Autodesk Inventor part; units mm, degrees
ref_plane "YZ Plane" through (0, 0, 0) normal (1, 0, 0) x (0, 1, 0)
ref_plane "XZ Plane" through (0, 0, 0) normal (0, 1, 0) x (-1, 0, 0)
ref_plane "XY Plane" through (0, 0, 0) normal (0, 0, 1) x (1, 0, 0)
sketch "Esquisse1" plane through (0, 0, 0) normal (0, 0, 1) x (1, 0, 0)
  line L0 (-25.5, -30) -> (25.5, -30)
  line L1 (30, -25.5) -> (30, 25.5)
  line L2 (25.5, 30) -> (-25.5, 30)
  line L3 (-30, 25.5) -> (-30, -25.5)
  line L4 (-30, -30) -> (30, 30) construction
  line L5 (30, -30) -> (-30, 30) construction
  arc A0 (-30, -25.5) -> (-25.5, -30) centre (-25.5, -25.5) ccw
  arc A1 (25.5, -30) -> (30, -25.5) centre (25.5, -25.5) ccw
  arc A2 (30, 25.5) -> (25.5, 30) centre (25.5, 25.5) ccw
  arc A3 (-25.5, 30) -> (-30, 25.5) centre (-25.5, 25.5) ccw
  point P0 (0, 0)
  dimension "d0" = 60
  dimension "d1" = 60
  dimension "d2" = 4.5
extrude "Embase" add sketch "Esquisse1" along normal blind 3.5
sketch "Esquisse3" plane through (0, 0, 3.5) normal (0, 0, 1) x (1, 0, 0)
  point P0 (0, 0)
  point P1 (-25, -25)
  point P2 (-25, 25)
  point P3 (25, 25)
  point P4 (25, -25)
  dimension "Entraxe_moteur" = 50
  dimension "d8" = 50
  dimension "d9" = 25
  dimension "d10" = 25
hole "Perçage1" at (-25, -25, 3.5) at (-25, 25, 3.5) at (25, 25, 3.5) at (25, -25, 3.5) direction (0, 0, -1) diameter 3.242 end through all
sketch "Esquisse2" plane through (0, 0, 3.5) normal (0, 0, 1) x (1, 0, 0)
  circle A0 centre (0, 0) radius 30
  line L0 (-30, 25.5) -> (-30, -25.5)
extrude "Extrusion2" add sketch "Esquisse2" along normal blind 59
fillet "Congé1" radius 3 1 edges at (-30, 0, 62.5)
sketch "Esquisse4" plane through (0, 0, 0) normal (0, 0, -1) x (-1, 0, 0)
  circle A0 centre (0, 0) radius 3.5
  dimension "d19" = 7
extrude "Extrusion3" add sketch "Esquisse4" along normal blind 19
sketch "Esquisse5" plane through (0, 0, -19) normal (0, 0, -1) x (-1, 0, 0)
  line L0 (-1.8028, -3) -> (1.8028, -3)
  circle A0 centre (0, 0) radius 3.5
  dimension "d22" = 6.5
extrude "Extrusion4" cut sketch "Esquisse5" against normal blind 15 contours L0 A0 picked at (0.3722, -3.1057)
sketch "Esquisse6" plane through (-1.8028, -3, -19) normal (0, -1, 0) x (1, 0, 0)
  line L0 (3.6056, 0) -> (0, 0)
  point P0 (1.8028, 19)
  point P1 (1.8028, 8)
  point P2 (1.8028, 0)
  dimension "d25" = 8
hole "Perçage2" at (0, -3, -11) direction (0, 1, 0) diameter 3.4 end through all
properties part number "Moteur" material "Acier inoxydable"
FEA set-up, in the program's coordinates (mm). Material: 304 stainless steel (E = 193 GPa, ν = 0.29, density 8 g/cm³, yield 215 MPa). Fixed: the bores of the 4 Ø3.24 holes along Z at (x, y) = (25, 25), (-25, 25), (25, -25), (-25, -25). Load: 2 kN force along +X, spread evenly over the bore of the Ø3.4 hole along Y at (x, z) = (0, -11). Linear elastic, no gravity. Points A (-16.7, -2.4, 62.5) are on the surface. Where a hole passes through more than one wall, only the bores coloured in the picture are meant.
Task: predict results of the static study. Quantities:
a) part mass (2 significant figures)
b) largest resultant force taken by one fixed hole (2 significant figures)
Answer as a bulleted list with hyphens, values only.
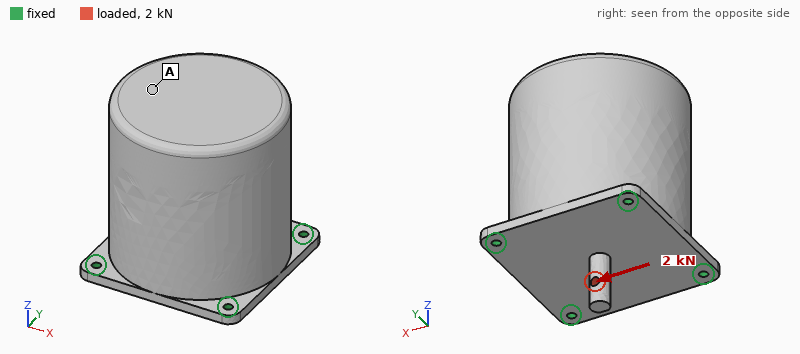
- 1.4 kg
- 580 N
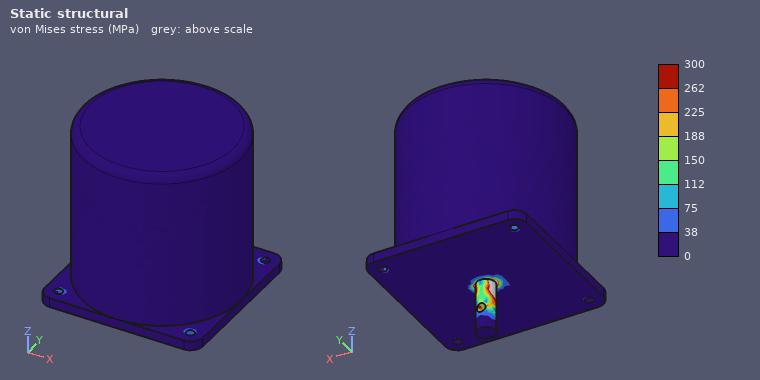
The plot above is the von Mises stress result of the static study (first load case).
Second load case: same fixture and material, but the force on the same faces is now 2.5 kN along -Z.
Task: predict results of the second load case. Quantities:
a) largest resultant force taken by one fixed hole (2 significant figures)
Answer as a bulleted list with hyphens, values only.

- 690 N
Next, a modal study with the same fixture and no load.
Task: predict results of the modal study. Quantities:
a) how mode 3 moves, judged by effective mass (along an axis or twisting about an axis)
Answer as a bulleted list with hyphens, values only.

- along Z
